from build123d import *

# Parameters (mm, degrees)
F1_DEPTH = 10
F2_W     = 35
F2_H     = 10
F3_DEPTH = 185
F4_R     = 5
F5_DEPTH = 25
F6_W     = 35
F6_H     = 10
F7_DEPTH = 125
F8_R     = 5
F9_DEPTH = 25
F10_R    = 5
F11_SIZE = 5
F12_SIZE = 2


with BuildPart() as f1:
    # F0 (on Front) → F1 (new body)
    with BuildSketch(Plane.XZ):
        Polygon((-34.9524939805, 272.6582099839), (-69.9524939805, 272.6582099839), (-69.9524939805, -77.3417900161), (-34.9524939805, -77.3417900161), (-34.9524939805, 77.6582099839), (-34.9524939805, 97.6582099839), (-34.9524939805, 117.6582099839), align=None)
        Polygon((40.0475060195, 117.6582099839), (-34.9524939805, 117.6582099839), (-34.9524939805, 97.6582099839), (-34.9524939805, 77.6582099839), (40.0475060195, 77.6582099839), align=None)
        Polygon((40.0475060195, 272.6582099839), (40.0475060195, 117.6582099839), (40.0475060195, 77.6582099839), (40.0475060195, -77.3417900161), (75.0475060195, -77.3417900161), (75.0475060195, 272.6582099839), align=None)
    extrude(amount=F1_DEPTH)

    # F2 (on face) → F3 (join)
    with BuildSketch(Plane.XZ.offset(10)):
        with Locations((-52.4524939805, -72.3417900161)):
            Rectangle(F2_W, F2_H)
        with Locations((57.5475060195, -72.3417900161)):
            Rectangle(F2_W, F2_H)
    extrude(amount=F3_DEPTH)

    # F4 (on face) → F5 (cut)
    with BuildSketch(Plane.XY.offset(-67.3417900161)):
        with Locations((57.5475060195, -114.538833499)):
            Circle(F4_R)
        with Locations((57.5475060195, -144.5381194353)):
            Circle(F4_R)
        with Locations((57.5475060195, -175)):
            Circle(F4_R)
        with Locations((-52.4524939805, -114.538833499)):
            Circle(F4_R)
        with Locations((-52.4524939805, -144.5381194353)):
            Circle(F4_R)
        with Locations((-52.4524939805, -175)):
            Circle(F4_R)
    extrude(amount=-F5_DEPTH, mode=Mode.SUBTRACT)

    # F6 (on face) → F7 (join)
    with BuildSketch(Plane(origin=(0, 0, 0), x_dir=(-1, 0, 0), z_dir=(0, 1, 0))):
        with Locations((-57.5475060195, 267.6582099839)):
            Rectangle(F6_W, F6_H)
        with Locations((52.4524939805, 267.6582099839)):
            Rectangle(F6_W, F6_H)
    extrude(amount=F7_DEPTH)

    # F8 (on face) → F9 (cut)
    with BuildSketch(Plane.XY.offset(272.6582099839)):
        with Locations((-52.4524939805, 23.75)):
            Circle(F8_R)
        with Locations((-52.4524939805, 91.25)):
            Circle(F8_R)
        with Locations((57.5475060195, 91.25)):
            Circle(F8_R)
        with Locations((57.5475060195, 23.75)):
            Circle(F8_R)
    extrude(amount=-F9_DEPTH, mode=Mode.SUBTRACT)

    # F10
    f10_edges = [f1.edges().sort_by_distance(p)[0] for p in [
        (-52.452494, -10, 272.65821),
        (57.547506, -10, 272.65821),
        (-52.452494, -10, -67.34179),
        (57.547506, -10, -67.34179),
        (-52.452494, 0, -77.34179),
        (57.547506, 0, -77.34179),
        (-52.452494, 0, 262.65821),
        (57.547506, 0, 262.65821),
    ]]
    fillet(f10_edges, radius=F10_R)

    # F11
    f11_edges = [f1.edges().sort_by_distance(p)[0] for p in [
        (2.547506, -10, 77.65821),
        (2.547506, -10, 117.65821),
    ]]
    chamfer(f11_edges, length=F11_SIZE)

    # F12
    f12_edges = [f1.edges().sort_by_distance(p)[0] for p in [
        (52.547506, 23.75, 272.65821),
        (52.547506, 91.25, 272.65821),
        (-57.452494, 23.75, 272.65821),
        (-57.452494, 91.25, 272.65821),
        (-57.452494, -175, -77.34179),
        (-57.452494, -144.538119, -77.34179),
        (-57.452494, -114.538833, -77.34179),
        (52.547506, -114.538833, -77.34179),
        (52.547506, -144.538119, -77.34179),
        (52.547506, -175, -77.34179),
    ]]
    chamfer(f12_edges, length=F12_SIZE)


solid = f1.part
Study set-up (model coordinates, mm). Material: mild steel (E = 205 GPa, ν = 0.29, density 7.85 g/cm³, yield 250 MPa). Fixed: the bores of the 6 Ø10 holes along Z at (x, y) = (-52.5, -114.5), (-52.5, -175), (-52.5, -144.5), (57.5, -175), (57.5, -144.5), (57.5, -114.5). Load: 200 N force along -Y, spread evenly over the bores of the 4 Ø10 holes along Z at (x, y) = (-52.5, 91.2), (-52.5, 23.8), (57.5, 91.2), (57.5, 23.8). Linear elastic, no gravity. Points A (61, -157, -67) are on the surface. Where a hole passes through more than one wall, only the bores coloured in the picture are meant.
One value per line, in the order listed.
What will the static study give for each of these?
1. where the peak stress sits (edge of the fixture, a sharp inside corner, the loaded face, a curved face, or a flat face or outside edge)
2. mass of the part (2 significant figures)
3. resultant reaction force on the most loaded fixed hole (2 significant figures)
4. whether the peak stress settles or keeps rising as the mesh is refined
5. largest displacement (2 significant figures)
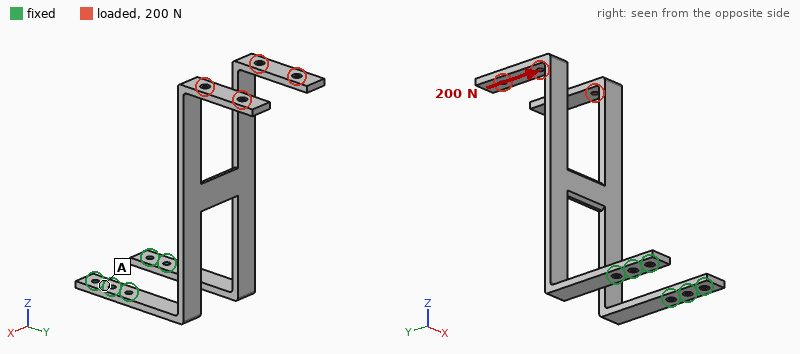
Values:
edge of the fixture
3.8 kg
370 N
keeps rising
4.8 mm
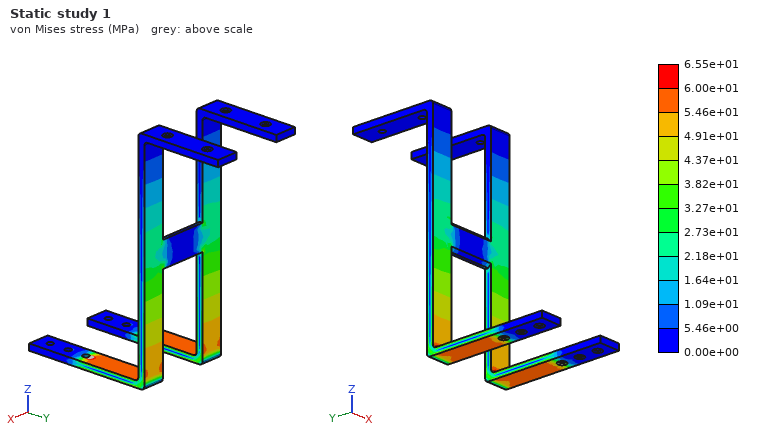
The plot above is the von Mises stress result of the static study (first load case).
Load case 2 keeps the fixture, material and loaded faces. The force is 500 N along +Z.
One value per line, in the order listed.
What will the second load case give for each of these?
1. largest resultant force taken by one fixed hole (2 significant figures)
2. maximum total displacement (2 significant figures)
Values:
630 N
4.0 mm
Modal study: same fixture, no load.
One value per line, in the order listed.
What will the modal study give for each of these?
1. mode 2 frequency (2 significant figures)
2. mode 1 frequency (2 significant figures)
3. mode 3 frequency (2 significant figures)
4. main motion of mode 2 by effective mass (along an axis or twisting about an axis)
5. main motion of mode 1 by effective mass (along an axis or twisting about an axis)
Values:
68 Hz
30 Hz
94 Hz
along X
along Y
